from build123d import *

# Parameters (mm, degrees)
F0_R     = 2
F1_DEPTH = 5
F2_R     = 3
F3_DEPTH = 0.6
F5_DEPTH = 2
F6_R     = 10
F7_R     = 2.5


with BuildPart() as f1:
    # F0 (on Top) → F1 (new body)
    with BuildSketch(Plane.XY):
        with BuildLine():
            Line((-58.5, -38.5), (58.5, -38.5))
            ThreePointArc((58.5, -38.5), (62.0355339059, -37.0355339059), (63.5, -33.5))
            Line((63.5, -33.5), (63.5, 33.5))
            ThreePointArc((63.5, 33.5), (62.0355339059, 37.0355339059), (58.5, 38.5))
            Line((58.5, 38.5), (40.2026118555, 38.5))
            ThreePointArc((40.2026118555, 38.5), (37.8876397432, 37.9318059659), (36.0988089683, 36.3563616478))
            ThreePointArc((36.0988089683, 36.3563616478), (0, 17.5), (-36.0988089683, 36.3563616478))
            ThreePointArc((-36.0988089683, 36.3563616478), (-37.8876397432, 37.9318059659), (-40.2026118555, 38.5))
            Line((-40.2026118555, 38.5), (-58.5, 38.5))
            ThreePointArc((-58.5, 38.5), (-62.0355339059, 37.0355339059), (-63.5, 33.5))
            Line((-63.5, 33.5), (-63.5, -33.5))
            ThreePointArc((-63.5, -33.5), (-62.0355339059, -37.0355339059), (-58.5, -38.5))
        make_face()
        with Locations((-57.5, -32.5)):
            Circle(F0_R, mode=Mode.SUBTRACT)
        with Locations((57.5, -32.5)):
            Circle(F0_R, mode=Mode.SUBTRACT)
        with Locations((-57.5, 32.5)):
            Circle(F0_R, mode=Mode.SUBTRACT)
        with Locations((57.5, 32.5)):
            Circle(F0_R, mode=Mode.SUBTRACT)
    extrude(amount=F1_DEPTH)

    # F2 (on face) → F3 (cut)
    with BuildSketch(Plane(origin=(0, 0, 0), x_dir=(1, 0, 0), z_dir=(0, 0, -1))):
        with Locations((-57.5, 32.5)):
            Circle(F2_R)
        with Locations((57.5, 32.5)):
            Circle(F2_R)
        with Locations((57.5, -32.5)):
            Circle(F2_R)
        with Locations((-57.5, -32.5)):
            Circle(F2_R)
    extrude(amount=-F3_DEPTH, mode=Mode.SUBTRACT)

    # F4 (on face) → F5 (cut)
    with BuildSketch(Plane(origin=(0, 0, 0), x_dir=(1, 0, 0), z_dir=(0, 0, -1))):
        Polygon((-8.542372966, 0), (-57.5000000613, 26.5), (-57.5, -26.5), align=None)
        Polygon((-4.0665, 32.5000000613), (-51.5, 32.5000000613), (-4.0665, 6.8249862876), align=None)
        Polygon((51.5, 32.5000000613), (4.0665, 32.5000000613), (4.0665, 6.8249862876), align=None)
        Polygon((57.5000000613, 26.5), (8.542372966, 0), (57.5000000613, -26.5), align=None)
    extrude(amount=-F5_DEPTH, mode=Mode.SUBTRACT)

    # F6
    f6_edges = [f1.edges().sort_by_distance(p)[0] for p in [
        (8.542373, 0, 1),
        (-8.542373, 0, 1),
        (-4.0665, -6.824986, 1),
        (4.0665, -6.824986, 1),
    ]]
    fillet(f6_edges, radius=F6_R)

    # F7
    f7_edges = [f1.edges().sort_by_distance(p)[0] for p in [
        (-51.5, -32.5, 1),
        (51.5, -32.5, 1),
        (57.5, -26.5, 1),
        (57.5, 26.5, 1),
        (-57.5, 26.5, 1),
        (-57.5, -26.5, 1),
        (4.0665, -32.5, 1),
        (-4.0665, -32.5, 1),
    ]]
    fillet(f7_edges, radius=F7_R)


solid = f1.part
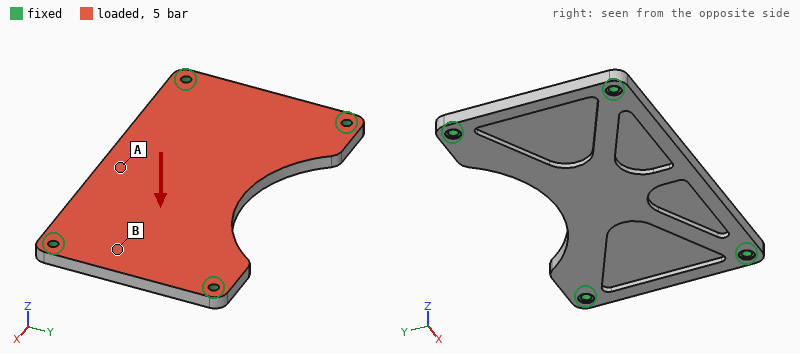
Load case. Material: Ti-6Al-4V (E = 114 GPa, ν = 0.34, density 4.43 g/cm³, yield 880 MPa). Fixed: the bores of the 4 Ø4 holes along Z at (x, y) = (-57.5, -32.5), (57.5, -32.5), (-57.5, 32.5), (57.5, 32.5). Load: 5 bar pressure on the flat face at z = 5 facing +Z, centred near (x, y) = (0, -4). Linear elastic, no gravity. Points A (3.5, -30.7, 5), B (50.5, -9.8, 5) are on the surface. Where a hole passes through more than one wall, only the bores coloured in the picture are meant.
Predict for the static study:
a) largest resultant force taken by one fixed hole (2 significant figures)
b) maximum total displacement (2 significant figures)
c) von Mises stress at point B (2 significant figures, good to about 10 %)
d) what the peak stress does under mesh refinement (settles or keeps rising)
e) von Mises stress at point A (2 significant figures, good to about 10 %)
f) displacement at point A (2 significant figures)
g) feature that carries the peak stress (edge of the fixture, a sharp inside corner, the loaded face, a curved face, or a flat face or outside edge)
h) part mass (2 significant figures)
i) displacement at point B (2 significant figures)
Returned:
1.3 kN
0.36 mm
40 MPa
keeps rising
95 MPa
0.36 mm
edge of the fixture
160 g
0.087 mm
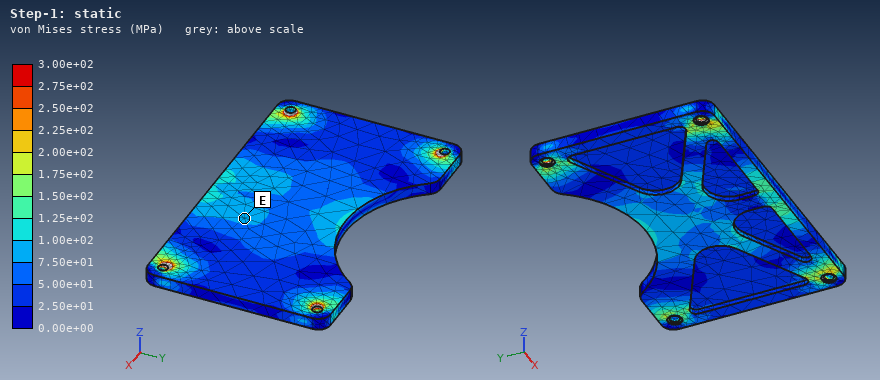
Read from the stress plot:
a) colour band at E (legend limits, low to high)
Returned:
7.50e+01 to 1.00e+02 MPa
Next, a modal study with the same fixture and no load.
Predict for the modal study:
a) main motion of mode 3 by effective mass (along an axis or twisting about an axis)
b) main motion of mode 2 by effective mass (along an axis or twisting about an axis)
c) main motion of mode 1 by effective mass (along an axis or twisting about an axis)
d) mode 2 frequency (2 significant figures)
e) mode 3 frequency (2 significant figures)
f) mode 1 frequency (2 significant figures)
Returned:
twisting about Y
twisting about X
along Z
2900 Hz
3900 Hz
1600 Hz
